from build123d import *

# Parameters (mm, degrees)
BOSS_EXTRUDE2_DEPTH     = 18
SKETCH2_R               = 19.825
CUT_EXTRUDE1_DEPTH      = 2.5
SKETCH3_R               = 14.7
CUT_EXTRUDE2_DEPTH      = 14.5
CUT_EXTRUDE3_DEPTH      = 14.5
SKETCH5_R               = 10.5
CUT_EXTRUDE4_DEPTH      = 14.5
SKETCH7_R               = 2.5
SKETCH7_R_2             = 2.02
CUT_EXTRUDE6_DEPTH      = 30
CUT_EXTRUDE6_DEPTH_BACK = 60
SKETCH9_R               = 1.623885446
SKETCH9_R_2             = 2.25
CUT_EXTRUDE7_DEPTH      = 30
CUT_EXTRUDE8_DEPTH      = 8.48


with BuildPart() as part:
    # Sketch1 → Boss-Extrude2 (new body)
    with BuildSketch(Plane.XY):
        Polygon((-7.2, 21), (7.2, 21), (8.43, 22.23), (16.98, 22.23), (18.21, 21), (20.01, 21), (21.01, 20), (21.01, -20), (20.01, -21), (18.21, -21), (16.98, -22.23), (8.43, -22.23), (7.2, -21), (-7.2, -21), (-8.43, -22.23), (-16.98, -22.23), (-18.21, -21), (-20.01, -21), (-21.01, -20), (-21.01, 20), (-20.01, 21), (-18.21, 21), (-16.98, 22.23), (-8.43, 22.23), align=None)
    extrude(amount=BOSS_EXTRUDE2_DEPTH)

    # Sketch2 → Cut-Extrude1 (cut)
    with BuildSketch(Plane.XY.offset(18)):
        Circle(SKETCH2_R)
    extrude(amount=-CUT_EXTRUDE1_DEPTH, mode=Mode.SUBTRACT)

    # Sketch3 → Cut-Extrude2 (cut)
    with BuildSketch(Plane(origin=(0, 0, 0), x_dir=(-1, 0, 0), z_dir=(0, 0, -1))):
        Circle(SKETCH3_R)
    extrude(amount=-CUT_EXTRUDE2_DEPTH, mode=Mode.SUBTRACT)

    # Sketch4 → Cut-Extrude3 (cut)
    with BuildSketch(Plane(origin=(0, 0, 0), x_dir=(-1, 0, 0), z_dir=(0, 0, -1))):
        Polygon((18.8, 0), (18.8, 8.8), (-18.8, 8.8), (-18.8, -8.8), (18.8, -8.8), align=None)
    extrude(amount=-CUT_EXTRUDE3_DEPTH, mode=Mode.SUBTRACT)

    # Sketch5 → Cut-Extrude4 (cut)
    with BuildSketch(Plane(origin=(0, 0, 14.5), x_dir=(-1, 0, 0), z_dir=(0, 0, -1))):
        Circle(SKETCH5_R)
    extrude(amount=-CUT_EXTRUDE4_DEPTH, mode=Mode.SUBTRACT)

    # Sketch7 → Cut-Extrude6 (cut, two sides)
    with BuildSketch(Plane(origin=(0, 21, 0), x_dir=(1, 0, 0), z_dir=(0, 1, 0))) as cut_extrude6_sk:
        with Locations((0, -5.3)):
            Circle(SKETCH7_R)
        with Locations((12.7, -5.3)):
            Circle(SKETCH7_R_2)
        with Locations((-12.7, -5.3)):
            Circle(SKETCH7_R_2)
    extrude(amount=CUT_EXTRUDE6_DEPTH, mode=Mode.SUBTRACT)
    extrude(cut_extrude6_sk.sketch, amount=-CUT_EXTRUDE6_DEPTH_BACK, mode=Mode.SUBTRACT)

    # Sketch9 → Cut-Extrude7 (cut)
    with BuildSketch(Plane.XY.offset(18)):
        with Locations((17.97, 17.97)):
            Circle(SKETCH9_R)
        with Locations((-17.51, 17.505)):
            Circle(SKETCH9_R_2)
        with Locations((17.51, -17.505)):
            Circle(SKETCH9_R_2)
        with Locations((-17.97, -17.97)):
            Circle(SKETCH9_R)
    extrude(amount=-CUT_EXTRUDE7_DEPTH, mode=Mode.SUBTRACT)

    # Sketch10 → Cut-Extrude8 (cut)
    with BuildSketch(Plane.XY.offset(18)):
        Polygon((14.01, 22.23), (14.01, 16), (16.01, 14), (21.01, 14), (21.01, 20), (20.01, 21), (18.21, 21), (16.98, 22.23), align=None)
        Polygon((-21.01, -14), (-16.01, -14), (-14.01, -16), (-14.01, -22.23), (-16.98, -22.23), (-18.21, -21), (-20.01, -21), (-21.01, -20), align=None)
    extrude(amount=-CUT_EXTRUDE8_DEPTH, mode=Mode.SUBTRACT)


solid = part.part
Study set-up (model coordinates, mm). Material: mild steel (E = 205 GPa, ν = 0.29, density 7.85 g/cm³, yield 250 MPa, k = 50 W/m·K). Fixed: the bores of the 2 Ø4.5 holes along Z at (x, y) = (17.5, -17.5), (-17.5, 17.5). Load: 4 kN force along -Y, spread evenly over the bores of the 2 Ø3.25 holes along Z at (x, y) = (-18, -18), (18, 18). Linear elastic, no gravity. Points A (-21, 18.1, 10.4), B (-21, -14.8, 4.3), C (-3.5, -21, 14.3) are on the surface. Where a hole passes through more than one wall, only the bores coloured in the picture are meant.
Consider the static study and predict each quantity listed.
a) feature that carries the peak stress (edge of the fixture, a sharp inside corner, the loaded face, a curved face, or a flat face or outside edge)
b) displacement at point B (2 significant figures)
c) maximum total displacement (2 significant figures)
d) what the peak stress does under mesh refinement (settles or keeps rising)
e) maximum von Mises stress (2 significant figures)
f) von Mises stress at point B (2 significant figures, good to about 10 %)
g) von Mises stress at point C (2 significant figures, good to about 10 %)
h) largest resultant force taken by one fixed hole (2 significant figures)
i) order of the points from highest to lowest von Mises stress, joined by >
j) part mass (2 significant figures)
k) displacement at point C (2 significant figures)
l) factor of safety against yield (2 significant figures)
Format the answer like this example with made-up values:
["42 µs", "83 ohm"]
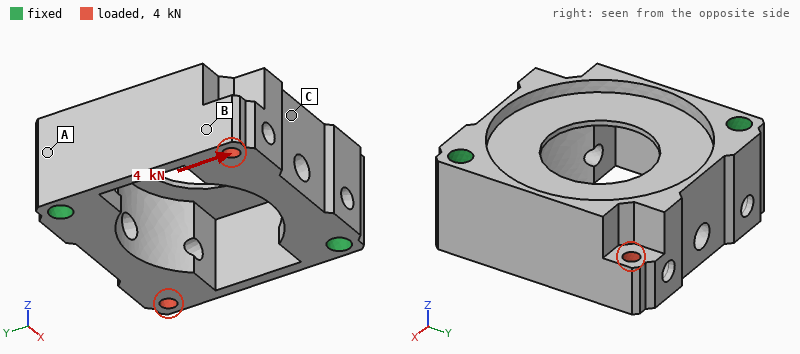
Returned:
["a flat face or outside edge", "9.5 µm", "13 µm", "settles", "98 MPa", "55 MPa", "20 MPa", "2.0 kN", "B > C > A", "110 g", "3.4 µm", "2.5"]
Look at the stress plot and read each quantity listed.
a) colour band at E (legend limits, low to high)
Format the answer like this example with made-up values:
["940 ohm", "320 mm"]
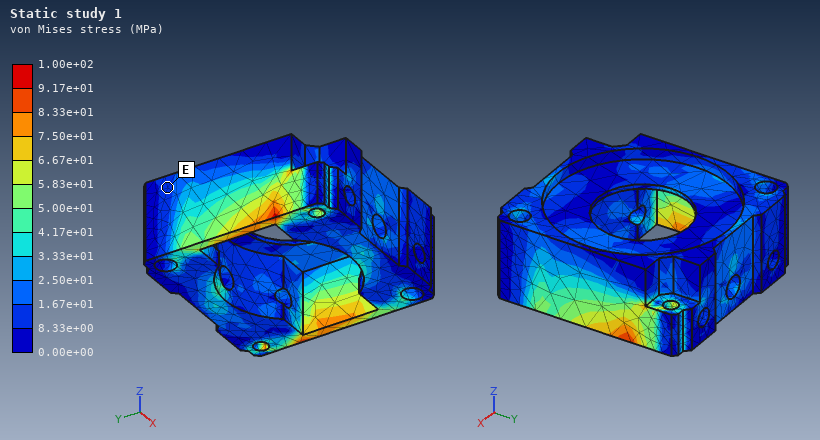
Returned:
["8.33e+00 to 1.67e+01 MPa"]
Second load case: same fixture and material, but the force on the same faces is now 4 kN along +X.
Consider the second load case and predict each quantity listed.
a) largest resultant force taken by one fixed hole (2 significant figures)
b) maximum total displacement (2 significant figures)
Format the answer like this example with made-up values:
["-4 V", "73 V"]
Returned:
["2.0 kN", "8.9 µm"]
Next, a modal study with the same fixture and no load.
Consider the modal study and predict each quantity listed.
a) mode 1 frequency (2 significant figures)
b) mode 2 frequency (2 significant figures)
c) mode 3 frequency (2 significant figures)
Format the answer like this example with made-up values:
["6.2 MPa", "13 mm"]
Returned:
["11 kHz", "11 kHz", "17 kHz"]
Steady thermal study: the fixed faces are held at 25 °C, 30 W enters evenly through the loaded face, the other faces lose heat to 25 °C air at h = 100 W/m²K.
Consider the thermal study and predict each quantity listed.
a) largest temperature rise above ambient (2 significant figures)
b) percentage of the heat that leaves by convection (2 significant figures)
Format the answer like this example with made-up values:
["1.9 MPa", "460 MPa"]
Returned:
["55 K", "48 %"]
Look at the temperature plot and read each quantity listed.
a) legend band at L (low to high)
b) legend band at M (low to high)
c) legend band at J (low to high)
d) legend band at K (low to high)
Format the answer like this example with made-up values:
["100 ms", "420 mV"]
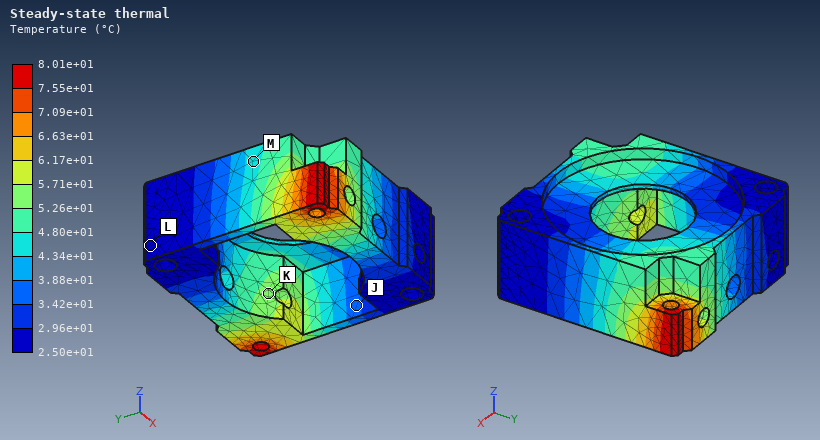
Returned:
["2.50e+01 to 2.96e+01 °C", "4.34e+01 to 4.80e+01 °C", "3.42e+01 to 3.88e+01 °C", "5.26e+01 to 5.71e+01 °C"]
